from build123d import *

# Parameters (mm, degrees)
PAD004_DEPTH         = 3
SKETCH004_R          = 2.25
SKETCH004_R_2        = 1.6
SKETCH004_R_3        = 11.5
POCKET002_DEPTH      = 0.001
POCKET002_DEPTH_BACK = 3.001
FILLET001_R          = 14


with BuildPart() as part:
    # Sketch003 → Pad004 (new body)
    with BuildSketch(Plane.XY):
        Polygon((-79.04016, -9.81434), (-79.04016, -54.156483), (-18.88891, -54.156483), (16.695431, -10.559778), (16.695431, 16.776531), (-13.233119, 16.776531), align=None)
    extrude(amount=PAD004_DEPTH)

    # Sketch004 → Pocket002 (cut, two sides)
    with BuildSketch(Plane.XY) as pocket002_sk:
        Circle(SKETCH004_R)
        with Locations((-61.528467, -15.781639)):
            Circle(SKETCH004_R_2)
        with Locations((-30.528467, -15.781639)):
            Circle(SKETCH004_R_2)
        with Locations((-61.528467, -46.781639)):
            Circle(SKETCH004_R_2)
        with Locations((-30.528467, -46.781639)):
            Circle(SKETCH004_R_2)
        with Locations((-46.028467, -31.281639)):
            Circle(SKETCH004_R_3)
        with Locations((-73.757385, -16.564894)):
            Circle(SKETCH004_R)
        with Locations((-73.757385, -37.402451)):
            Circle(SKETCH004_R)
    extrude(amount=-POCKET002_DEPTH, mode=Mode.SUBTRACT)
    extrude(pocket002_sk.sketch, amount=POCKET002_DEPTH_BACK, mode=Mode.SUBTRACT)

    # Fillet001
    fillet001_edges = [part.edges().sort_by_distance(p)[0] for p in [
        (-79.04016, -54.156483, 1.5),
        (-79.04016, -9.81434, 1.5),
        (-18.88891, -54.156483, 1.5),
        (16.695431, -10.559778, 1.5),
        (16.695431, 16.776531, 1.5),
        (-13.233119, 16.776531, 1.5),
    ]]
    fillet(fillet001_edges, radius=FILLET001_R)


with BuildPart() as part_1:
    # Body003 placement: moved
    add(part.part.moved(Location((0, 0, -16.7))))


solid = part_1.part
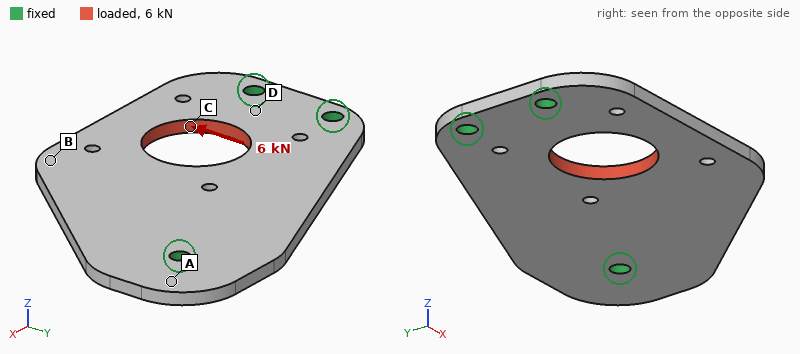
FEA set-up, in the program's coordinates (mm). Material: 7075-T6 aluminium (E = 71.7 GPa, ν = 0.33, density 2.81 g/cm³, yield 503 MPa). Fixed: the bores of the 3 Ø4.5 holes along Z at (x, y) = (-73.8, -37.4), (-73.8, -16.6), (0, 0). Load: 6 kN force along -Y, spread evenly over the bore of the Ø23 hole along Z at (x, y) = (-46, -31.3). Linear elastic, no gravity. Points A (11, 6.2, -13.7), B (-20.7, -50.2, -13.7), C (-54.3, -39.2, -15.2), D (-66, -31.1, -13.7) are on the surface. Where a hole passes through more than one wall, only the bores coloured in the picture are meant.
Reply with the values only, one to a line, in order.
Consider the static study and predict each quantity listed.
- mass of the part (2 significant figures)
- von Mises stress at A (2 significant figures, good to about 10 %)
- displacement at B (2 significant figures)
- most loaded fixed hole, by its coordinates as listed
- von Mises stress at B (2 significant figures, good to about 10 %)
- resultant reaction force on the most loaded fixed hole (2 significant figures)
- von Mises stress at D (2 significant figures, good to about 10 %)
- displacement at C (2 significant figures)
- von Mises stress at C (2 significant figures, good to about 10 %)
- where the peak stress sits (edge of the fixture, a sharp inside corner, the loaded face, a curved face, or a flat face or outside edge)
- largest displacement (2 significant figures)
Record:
38 g
11 MPa
31 µm
(0, 0)
21 MPa
2.4 kN
74 MPa
30 µm
88 MPa
edge of the fixture
44 µm
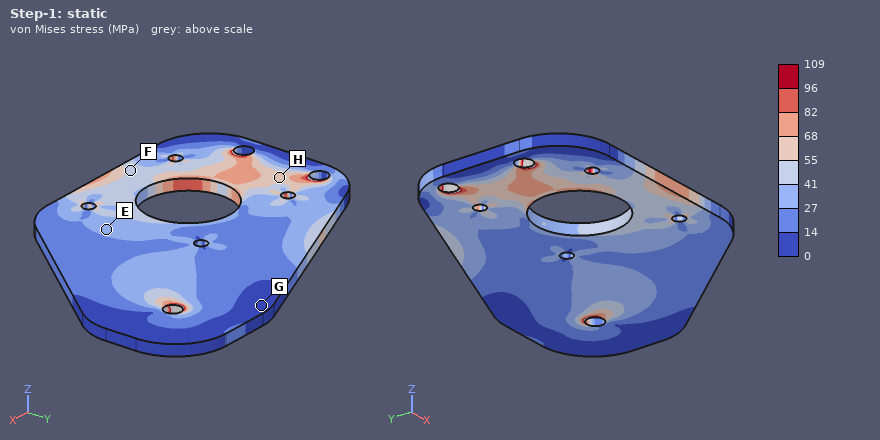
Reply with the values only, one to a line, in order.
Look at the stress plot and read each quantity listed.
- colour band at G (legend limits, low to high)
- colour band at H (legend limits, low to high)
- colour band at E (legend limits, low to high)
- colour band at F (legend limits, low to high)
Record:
0 to 14 MPa
55 to 68 MPa
27 to 41 MPa
41 to 55 MPa
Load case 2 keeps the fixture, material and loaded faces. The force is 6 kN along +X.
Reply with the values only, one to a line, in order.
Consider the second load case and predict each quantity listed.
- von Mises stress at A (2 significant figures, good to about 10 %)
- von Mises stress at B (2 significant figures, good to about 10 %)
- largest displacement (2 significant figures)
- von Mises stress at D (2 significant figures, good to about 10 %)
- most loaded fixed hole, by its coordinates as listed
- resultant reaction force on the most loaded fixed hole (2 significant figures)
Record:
11 MPa
16 MPa
35 µm
26 MPa
(-73.8, -37.4)
2.6 kN
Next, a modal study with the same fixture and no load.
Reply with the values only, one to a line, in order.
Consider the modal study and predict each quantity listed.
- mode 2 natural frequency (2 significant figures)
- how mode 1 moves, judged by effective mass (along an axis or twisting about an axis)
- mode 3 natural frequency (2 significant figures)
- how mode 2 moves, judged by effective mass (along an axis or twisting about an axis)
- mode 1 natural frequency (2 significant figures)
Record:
2800 Hz
along Z
4000 Hz
along Z
1400 Hz
